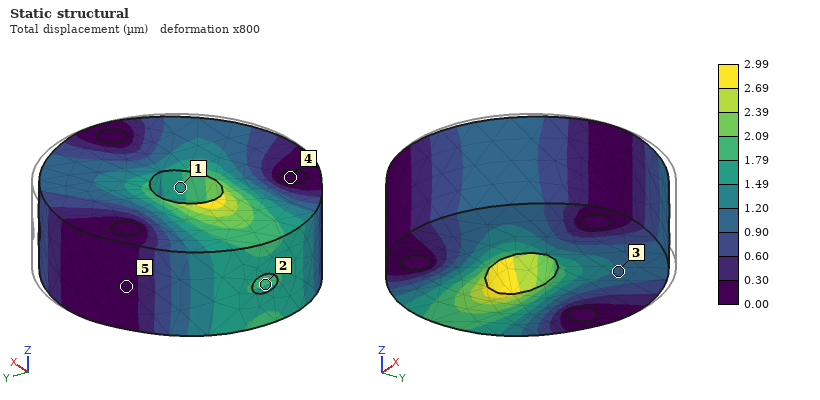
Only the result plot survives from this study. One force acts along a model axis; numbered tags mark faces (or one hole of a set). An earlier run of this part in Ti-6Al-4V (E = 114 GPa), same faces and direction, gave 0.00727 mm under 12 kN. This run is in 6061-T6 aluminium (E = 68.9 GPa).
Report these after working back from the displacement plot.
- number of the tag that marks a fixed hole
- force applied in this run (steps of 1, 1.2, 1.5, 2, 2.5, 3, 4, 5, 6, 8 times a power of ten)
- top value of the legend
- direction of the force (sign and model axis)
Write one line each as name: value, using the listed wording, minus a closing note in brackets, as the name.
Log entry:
number of the tag that marks a fixed hole: 4
force applied in this run: 3 kN
top value of the legend: 2.99 µm
direction of the force: -X
